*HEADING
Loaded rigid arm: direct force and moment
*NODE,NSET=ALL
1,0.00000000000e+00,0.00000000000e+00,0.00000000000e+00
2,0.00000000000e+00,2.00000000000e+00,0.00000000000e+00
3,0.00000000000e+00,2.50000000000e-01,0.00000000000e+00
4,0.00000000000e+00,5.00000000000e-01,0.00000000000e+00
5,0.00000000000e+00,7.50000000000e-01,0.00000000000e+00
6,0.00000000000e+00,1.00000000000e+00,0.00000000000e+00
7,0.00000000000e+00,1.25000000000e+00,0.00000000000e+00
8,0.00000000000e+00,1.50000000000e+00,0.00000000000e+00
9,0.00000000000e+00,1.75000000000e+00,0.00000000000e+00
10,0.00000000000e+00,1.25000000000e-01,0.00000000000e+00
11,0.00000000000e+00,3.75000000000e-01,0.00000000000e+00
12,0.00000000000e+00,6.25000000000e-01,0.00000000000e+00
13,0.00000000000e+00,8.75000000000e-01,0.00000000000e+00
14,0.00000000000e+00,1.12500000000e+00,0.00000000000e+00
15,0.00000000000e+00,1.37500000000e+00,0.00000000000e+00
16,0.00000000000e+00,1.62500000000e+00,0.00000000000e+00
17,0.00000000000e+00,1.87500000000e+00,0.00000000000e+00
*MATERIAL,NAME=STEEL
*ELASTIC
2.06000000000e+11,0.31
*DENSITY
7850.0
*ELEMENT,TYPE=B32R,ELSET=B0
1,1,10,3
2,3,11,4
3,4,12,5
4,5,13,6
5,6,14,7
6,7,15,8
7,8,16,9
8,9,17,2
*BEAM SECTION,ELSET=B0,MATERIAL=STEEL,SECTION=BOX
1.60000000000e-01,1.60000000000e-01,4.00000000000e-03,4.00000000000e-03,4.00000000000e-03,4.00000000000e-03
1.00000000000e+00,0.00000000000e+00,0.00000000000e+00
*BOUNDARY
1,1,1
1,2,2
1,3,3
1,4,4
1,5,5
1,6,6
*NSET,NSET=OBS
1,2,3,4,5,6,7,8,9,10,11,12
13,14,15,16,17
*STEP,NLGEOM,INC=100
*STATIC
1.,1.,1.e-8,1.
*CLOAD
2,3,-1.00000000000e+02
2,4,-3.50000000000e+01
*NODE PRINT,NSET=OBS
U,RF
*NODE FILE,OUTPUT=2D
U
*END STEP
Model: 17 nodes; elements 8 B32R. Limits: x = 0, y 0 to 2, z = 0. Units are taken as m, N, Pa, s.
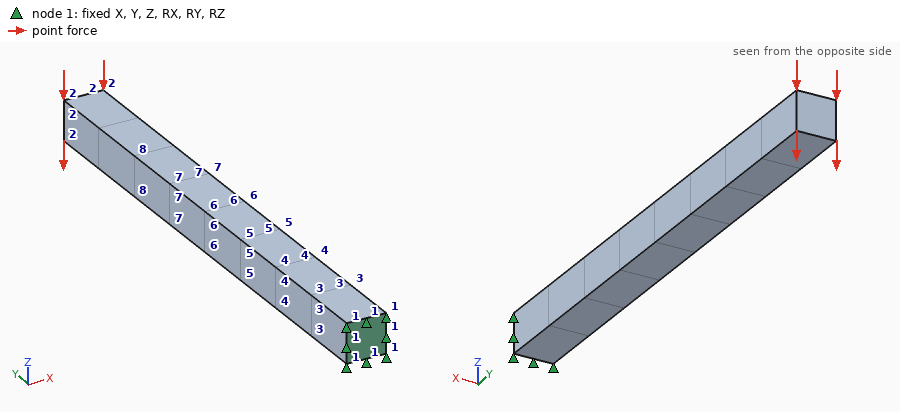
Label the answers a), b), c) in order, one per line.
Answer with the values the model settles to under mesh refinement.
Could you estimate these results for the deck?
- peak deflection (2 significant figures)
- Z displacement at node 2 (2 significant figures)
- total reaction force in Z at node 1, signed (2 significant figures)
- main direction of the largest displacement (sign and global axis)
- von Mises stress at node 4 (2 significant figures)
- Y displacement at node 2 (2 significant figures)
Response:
a) 1.6e-04 m
b) -1.6e-04 m
c) 100 N
d) -Z
e) 1.5e+06 Pa
f) 1.0e-05 m
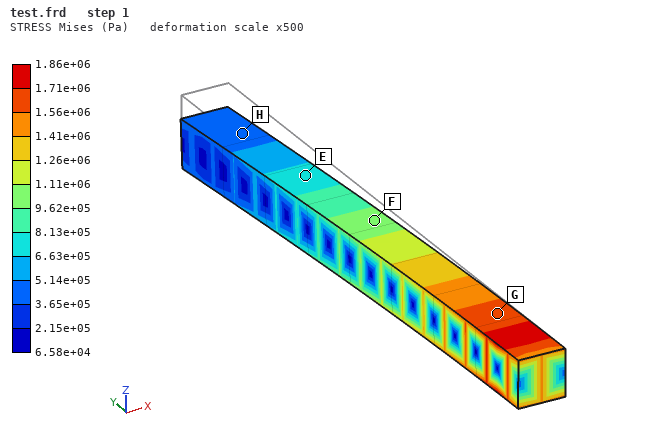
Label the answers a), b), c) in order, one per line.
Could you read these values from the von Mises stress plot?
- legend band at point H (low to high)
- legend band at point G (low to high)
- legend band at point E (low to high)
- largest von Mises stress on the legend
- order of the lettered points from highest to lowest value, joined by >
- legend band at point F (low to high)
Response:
a) 3.65e+05 to 5.14e+05 Pa
b) 1.56e+06 to 1.71e+06 Pa
c) 6.63e+05 to 8.13e+05 Pa
d) 1.86e+06 Pa
e) G > F > E > H
f) 9.62e+05 to 1.11e+06 Pa
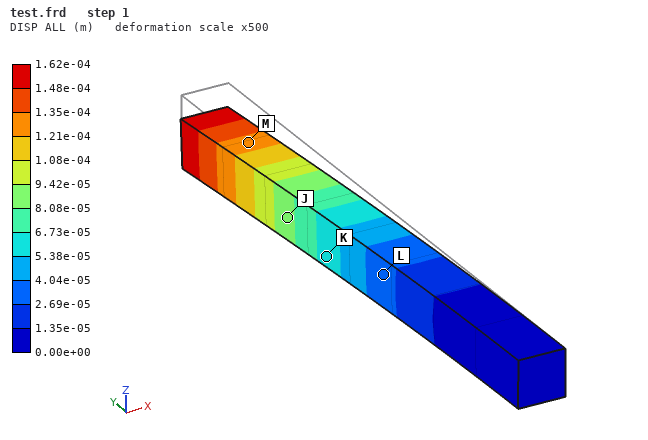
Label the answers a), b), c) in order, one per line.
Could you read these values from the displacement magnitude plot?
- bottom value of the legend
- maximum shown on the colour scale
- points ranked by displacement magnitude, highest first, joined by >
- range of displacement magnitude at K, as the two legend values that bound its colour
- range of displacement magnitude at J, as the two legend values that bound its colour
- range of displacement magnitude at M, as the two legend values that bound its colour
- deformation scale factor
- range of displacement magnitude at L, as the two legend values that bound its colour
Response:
a) 0.00e+00 m
b) 1.62e-04 m
c) M > J > K > L
d) 5.38e-05 to 6.73e-05 m
e) 8.08e-05 to 9.42e-05 m
f) 1.21e-04 to 1.35e-04 m
g) 500
h) 2.69e-05 to 4.04e-05 m
